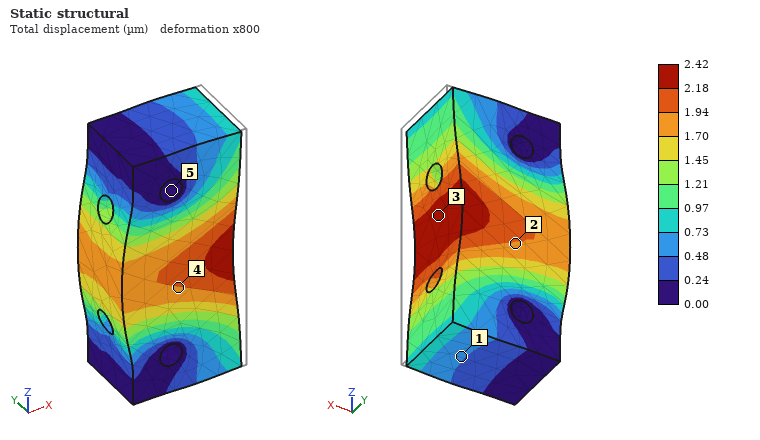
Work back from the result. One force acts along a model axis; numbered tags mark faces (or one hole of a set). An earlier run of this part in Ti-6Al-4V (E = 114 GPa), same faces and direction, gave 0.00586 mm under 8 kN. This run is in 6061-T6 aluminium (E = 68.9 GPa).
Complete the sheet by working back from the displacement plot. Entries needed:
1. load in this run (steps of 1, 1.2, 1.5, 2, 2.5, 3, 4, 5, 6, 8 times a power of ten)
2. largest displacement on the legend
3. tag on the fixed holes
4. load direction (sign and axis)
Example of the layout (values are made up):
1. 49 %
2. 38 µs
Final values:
1. 2 kN
2. 2.42 µm
3. 5
4. -X
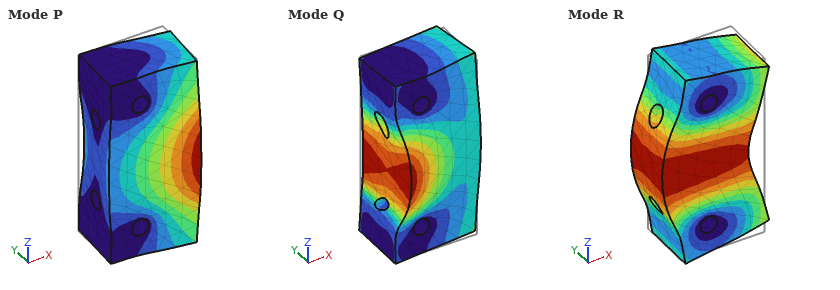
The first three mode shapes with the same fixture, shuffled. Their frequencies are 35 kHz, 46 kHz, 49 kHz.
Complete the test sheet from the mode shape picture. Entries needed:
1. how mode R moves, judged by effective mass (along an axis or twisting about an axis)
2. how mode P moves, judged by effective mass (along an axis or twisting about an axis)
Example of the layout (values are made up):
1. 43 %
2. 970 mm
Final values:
1. along X
2. along Y
